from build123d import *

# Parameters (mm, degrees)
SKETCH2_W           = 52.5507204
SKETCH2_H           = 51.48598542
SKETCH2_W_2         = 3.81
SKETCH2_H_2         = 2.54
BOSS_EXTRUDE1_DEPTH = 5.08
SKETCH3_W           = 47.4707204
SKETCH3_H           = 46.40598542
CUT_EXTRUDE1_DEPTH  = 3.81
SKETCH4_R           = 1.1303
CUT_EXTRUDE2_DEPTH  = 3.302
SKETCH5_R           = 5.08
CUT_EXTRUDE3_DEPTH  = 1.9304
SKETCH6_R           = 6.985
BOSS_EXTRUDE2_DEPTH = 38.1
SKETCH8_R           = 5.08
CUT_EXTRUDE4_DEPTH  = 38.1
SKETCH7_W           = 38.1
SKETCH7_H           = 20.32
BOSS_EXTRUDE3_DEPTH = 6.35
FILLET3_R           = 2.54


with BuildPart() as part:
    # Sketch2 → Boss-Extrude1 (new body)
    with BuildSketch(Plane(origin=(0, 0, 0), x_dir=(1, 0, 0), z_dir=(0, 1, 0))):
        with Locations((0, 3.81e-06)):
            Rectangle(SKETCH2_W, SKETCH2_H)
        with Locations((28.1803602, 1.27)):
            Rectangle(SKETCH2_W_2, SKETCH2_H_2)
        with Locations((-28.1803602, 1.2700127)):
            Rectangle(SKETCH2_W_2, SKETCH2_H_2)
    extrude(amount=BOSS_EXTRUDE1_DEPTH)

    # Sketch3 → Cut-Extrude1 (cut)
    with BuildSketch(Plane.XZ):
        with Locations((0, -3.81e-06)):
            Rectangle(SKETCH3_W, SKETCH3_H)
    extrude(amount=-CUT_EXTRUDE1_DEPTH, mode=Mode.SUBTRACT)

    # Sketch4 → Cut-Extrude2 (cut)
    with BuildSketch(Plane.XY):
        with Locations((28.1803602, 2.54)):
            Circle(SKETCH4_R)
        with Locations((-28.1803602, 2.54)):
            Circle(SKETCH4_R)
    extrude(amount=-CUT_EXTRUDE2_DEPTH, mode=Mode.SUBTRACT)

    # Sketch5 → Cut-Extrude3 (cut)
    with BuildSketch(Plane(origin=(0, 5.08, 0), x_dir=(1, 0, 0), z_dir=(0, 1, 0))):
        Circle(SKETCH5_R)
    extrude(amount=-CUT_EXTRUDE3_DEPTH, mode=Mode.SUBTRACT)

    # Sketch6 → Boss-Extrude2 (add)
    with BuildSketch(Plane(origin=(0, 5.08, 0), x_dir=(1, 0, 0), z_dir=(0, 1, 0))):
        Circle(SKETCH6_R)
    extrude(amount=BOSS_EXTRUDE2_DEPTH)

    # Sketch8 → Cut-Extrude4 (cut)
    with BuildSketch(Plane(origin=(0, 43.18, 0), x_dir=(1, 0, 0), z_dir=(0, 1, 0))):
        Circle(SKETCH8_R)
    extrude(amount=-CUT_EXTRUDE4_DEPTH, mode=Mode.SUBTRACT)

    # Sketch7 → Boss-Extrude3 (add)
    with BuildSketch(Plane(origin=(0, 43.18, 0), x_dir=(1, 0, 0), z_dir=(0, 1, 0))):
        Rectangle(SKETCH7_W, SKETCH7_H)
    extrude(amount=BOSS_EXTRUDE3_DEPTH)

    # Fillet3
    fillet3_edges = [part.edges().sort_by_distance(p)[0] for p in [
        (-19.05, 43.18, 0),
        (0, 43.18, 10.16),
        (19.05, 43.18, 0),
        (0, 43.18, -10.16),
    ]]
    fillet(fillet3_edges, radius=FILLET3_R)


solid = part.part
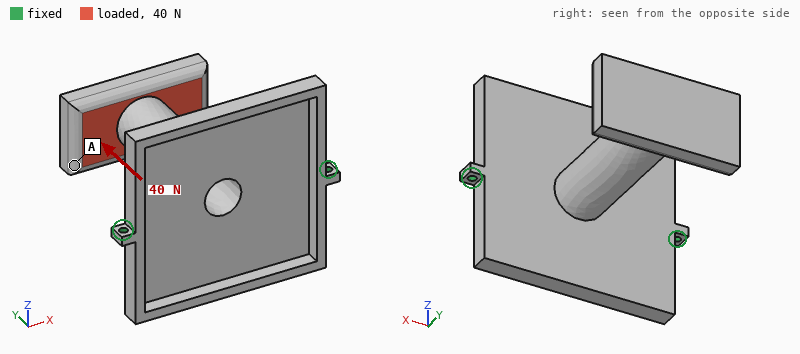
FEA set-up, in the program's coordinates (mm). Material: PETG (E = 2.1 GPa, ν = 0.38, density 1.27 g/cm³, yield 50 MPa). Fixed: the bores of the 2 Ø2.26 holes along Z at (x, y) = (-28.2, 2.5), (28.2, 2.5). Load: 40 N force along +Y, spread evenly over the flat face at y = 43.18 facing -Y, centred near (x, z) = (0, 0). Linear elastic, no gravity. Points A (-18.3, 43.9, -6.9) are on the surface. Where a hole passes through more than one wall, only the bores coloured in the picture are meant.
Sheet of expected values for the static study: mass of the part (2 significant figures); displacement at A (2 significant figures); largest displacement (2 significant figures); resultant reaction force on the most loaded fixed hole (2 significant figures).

16 g
0.87 mm
0.95 mm
36 N
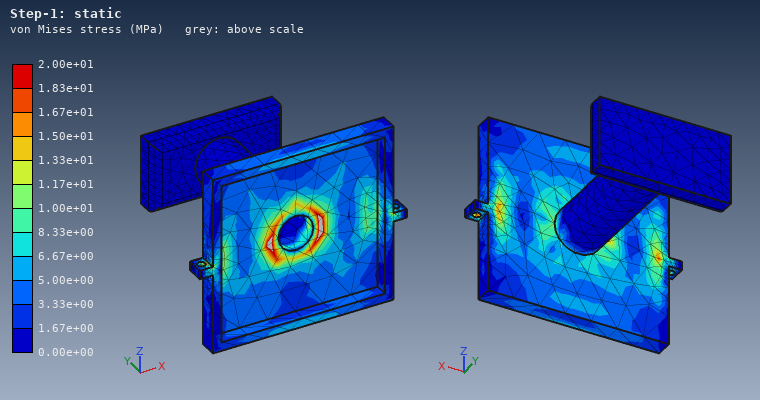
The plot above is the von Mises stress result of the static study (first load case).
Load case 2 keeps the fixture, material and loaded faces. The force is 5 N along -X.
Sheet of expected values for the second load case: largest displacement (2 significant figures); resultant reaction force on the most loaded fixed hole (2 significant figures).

1.1 mm
5.4 N
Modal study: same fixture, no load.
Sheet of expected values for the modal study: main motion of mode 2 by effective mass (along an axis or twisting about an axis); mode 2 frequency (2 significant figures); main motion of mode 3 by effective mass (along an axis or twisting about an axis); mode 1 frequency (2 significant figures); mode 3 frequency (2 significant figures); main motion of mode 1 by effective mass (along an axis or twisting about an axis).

along X
130 Hz
along Y
96 Hz
330 Hz
along Z
